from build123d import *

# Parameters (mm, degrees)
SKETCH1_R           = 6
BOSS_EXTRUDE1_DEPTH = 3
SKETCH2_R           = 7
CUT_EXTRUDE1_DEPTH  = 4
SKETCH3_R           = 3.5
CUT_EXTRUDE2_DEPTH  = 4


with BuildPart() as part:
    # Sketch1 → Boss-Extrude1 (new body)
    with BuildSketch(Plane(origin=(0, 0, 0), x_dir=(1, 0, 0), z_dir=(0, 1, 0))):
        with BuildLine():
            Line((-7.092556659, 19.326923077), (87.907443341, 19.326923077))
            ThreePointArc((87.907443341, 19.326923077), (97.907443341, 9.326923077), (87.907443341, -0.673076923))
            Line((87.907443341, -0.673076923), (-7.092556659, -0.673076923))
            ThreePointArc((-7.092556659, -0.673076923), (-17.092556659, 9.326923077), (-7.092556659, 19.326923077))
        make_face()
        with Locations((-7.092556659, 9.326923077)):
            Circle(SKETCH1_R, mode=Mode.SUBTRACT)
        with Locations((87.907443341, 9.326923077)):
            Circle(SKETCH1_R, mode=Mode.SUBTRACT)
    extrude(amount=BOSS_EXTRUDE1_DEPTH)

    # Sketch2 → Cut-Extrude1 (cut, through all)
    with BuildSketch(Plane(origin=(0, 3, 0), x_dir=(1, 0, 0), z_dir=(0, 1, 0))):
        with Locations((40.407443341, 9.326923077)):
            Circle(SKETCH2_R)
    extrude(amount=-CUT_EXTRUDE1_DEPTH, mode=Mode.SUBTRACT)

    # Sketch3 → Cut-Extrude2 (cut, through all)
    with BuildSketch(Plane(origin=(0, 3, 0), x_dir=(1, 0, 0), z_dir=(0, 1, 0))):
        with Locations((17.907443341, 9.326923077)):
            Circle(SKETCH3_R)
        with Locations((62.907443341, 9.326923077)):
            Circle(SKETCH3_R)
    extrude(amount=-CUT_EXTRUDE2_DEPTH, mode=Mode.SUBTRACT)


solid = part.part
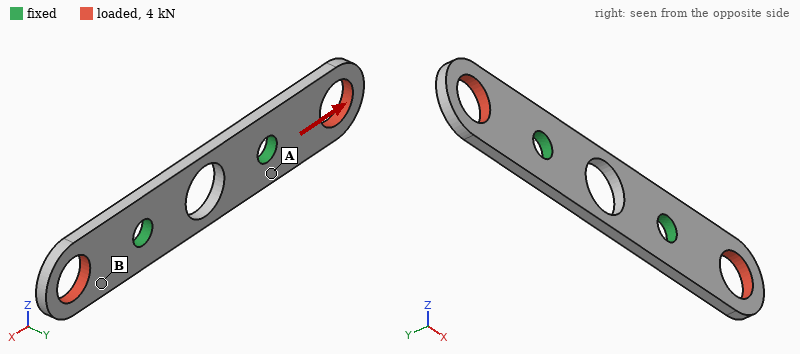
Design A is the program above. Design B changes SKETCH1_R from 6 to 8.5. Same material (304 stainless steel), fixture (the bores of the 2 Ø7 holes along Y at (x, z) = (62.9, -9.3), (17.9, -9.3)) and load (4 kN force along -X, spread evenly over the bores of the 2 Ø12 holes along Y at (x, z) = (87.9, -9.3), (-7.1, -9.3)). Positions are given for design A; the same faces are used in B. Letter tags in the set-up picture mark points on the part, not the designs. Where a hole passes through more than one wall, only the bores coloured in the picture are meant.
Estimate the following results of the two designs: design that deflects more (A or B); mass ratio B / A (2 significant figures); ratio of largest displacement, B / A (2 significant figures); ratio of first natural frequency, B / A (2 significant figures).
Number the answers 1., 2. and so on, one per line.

1. B
2. 0.87
3. 5.8
4. 1.3
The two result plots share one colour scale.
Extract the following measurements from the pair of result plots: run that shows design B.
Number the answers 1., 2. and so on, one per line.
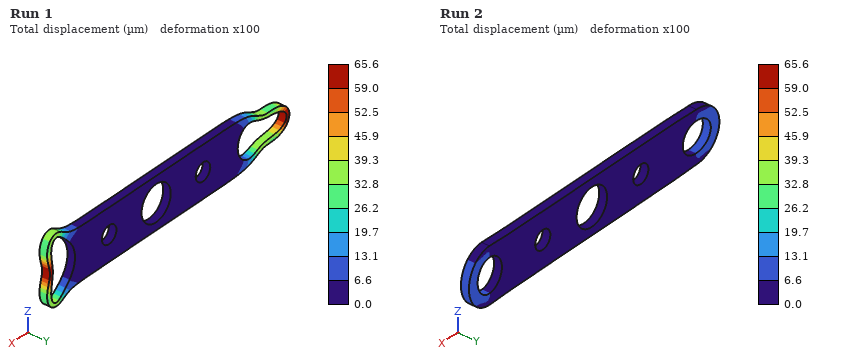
1. Run 1
